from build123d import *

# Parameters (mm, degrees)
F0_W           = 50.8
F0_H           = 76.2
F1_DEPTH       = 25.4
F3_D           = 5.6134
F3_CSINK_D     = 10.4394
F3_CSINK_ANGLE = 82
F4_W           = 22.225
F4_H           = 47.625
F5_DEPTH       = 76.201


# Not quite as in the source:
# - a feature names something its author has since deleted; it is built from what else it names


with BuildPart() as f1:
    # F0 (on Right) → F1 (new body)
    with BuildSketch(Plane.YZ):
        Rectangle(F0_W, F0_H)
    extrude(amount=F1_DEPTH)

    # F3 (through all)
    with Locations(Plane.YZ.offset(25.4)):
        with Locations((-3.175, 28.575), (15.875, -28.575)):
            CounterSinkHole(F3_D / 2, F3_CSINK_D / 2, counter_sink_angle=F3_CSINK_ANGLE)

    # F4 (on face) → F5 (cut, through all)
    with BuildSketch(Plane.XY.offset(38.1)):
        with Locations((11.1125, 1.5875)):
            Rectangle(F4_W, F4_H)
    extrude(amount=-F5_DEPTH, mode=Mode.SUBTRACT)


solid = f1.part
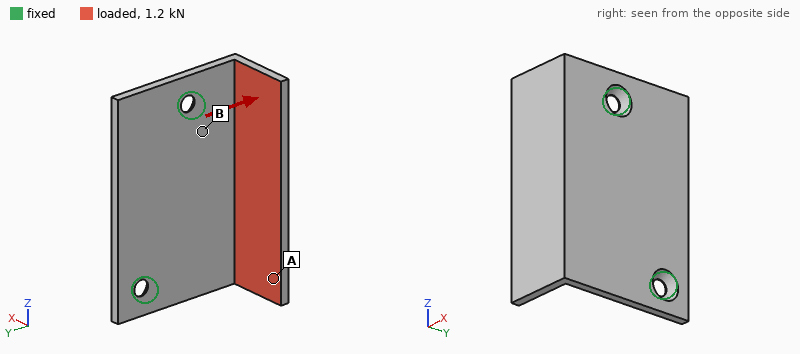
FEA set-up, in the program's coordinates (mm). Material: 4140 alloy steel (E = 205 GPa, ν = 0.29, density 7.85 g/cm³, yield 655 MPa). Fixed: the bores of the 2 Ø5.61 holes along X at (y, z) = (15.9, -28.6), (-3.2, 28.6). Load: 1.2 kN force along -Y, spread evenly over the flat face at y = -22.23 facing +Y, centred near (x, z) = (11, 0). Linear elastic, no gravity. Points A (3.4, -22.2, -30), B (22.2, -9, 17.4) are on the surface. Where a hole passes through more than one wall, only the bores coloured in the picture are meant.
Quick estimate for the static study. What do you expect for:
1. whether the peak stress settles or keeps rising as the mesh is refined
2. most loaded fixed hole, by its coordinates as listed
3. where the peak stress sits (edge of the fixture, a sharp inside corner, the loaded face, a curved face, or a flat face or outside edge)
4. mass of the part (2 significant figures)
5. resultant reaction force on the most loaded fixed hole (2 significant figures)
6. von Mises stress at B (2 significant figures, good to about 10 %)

keeps rising
(-3.2, 28.6)
edge of the fixture
140 g
650 N
130 MPa
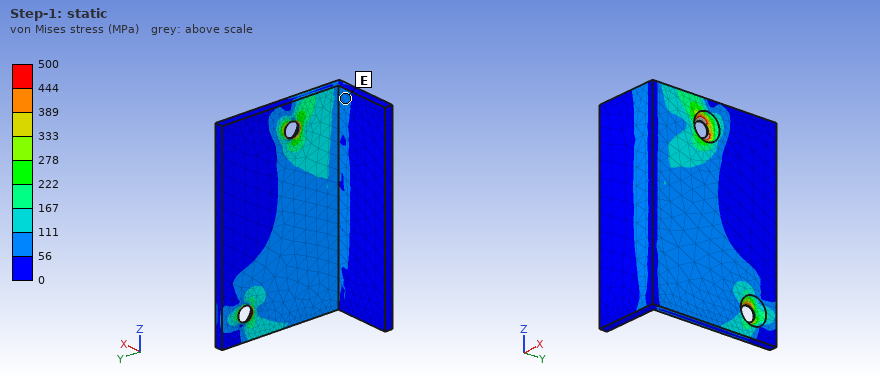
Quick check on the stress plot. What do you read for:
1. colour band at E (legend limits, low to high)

56 to 111 MPa
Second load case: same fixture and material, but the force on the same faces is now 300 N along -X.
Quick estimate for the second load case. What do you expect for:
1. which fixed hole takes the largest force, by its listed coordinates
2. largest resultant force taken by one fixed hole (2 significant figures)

(-3.2, 28.6)
250 N
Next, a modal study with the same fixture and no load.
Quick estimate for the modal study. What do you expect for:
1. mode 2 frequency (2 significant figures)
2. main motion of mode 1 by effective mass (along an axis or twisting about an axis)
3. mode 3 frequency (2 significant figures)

1800 Hz
along X
2700 Hz
